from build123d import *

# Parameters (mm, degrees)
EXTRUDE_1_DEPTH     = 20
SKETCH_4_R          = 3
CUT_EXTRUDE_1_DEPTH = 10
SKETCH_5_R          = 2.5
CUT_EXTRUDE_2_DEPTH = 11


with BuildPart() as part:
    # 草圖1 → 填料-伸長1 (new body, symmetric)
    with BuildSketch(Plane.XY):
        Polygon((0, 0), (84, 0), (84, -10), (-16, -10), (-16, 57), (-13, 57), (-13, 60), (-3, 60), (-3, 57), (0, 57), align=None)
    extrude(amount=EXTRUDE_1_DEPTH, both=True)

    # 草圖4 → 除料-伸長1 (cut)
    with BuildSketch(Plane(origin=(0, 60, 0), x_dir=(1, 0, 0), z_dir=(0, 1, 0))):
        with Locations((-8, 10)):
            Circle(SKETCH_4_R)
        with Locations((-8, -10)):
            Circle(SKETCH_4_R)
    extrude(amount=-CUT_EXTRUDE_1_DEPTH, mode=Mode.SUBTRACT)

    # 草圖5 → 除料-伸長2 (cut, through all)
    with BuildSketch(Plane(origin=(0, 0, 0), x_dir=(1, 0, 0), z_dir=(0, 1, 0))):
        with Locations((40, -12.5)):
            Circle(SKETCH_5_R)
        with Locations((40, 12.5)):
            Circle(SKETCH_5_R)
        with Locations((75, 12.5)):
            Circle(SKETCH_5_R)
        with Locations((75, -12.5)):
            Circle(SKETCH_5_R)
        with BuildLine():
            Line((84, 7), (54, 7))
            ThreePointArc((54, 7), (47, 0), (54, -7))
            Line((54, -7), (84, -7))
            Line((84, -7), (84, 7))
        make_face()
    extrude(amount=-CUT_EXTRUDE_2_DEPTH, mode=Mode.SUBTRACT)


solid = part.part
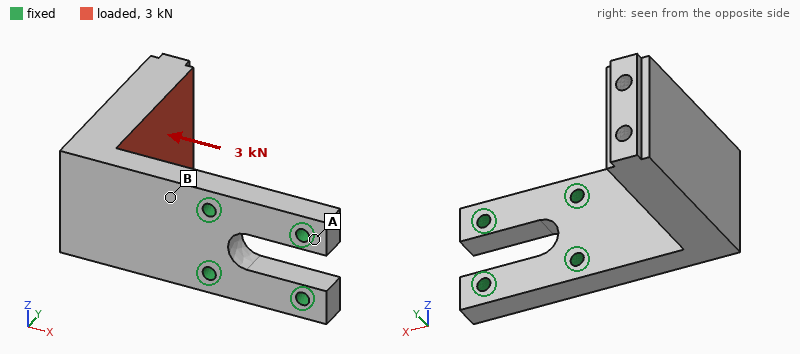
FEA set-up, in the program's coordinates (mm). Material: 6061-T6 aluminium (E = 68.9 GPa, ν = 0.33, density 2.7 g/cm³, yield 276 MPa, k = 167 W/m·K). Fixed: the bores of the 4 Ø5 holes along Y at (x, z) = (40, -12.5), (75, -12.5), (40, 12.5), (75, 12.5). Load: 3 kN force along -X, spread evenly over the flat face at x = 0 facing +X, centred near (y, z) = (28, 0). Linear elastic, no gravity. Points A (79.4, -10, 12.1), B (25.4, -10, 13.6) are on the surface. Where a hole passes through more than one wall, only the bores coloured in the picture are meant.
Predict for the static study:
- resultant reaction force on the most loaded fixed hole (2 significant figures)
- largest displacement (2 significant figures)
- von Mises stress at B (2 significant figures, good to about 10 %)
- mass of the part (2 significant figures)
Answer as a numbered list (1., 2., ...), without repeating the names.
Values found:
1. 1.5 kN
2. 1.5 mm
3. 140 MPa
4. 190 g
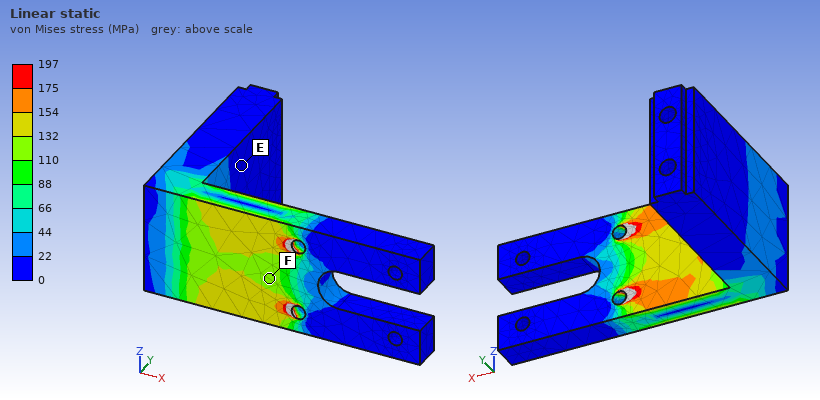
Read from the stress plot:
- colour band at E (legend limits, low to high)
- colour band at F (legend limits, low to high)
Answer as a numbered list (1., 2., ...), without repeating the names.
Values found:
1. 0 to 22 MPa
2. 110 to 132 MPa
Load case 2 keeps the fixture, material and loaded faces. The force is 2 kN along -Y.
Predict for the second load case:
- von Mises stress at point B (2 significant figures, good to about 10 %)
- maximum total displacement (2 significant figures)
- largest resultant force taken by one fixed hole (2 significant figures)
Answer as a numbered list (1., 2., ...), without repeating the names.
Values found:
1. 77 MPa
2. 0.52 mm
3. 1.2 kN
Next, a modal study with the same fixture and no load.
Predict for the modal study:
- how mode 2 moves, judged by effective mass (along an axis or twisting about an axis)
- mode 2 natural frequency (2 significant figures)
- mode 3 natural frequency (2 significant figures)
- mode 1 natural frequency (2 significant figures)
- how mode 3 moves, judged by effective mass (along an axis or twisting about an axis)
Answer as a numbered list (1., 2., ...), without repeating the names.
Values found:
1. along Z
2. 1200 Hz
3. 2600 Hz
4. 730 Hz
5. along Y
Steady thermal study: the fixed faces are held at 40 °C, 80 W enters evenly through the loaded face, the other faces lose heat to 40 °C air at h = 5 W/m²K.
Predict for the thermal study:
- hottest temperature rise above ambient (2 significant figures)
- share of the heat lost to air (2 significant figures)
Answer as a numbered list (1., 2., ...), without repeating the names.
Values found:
1. 75 K
2. 3.4 %
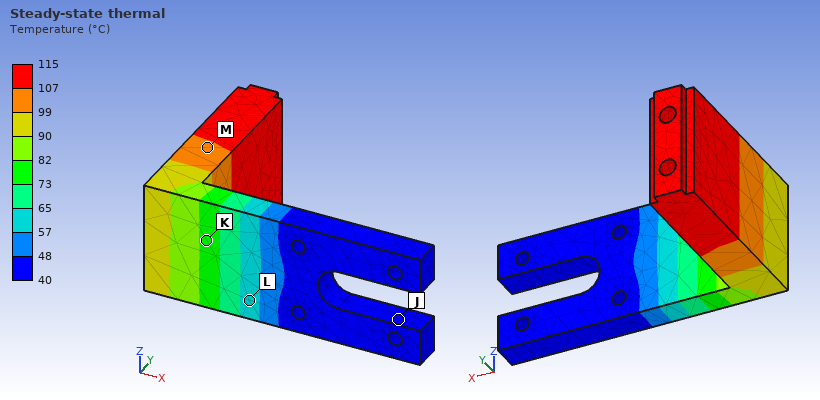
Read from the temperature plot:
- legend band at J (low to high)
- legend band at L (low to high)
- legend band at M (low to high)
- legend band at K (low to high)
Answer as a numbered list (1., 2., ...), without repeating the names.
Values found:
1. 40 to 48 °C
2. 57 to 65 °C
3. 99 to 107 °C
4. 73 to 82 °C
